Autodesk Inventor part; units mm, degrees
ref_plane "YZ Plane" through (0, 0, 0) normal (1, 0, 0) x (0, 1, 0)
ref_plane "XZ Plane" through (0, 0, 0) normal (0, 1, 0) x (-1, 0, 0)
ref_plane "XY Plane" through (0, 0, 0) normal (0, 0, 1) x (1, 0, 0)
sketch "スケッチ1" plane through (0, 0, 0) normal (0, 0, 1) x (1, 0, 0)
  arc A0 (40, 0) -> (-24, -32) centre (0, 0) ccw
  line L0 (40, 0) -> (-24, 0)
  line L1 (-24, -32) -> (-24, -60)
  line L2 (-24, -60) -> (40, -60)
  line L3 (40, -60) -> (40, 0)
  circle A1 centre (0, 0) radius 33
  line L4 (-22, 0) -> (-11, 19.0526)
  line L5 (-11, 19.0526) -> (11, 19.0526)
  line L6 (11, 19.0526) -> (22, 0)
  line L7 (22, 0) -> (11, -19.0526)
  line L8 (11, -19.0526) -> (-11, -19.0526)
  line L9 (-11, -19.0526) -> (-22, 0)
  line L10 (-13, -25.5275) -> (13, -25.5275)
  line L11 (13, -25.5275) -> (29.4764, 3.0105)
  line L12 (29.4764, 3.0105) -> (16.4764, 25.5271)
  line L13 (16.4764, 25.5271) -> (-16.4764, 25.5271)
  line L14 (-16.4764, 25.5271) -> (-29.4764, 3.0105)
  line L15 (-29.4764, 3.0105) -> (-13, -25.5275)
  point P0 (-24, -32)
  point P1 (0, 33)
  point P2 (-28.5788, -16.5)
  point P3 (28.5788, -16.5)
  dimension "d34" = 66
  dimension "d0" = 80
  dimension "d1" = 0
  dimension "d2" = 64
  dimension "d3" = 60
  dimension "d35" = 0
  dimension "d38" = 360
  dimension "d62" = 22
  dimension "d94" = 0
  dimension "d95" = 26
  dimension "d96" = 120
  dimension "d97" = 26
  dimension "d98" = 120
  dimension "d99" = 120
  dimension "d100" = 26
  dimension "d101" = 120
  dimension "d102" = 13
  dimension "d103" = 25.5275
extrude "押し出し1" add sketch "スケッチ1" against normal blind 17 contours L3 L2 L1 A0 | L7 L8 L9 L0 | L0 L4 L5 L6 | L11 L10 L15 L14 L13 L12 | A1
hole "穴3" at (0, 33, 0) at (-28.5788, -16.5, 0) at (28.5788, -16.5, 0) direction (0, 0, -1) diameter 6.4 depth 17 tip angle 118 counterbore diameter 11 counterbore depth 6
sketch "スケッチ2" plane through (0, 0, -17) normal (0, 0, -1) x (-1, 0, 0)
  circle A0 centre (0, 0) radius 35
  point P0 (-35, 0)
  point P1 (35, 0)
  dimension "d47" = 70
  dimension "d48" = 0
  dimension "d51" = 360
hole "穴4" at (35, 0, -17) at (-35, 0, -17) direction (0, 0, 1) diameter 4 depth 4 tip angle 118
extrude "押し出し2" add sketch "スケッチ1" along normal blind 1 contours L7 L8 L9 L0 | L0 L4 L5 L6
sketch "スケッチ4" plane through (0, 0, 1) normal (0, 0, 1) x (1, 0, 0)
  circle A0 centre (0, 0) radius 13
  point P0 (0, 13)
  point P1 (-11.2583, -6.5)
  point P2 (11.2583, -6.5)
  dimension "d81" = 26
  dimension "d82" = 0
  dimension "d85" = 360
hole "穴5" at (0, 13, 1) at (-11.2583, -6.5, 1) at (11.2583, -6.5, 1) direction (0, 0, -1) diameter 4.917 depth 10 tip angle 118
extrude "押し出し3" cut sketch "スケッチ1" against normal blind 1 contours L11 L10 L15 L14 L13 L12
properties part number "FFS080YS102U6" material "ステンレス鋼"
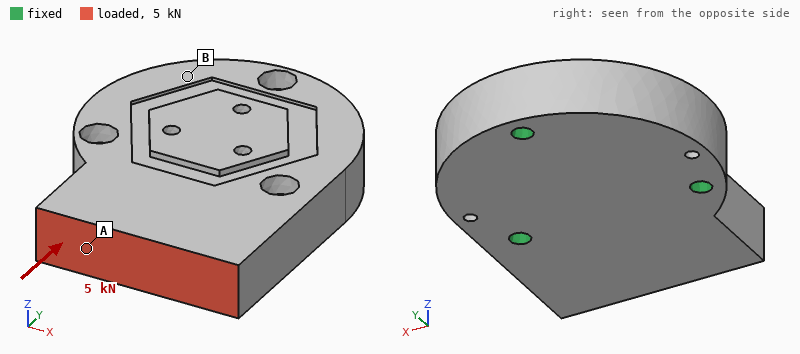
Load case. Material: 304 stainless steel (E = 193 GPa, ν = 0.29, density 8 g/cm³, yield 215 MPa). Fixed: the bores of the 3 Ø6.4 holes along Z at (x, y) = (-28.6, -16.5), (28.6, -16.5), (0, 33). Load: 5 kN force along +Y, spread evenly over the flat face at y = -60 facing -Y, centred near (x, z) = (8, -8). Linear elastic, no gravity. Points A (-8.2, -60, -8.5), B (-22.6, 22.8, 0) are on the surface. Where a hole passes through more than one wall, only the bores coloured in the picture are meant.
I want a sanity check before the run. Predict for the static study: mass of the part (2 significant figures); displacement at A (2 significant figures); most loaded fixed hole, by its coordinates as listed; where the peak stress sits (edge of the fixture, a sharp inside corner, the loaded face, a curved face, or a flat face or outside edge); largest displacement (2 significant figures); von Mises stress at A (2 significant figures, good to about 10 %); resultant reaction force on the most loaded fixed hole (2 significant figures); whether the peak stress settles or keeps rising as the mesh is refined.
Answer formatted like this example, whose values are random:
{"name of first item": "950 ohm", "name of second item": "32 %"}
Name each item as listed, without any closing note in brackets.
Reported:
{"mass of the part": "890 g", "displacement at A": "2.0 µm", "most loaded fixed hole, by its coordinates as listed": "(28.6, -16.5)", "where the peak stress sits": "edge of the fixture", "largest displacement": "2.4 µm", "von Mises stress at A": "4.4 MPa", "resultant reaction force on the most loaded fixed hole": "2.7 kN", "whether the peak stress settles or keeps rising as the mesh is refined": "keeps rising"}
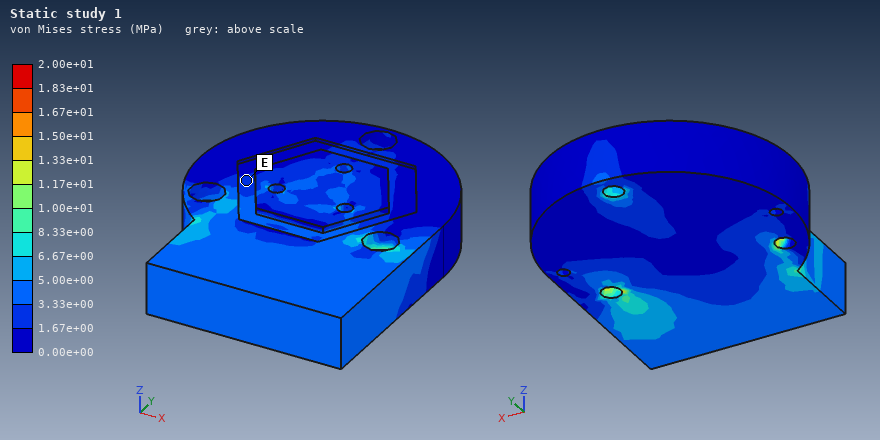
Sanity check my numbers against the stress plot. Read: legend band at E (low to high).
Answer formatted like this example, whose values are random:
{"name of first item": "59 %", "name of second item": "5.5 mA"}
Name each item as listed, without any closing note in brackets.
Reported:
{"legend band at E": "1.67e+00 to 3.33e+00 MPa"}
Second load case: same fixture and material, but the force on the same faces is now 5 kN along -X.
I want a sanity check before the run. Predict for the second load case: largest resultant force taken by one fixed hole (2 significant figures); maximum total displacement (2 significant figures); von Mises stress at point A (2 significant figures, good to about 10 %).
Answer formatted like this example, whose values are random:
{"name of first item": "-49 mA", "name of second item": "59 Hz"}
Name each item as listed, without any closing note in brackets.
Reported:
{"largest resultant force taken by one fixed hole": "4.5 kN", "maximum total displacement": "7.0 µm", "von Mises stress at point A": "10 MPa"}
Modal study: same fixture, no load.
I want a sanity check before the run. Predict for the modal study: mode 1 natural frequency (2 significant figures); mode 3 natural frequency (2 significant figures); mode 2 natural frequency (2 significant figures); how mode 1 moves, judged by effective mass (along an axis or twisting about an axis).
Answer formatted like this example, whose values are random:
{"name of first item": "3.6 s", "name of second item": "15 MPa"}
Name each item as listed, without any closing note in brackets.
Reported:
{"mode 1 natural frequency": "4600 Hz", "mode 3 natural frequency": "11 kHz", "mode 2 natural frequency": "9500 Hz", "how mode 1 moves, judged by effective mass": "along Z"}
